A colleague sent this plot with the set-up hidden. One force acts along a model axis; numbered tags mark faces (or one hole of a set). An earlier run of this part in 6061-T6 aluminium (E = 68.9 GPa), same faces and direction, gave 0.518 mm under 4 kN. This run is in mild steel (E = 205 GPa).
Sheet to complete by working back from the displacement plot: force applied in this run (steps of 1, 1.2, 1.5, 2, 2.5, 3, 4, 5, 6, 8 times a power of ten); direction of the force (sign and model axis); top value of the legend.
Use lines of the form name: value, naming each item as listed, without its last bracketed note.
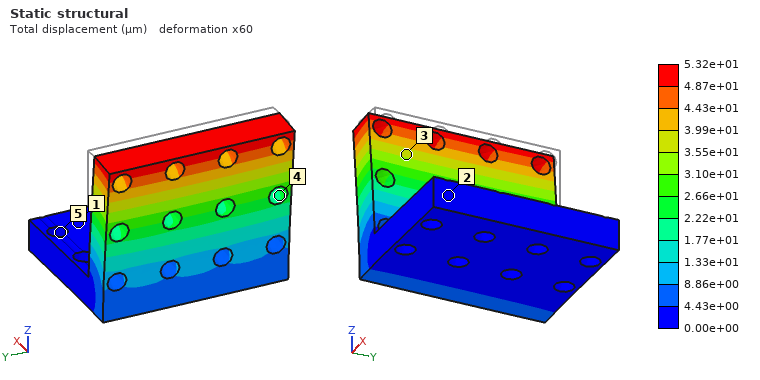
force applied in this run: 1.2 kN
direction of the force: -X
top value of the legend: 5.32e+01 µm
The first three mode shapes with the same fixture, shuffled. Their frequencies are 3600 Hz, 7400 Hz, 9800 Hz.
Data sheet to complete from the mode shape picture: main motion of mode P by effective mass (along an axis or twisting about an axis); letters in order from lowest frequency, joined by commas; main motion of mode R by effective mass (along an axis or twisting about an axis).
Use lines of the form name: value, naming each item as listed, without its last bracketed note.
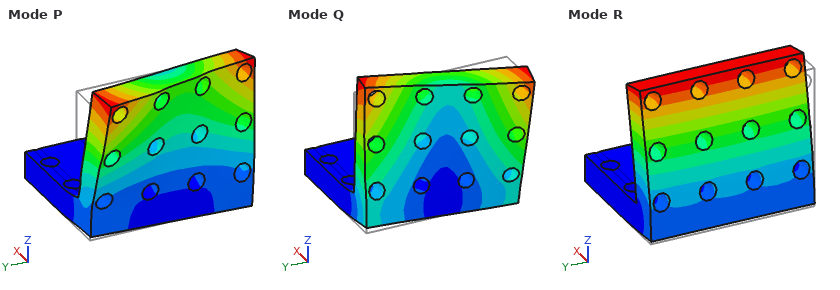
main motion of mode P by effective mass: along Y
letters in order from lowest frequency, joined by commas: R, Q, P
main motion of mode R by effective mass: along X
